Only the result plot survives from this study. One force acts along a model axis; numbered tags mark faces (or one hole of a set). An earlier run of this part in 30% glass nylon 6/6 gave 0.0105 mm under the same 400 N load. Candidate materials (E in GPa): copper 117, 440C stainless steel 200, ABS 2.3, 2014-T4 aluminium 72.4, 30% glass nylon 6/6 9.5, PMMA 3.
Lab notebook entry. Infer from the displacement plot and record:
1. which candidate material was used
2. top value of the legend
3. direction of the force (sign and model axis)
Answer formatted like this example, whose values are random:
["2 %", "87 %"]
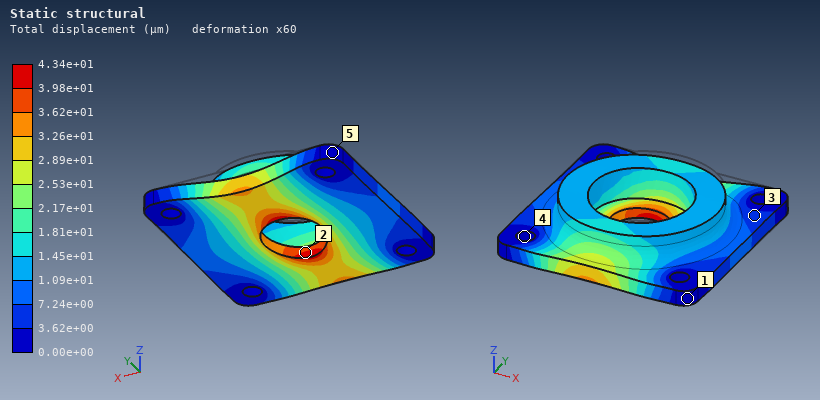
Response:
["ABS", "4.34e+01 µm", "-Y"]
